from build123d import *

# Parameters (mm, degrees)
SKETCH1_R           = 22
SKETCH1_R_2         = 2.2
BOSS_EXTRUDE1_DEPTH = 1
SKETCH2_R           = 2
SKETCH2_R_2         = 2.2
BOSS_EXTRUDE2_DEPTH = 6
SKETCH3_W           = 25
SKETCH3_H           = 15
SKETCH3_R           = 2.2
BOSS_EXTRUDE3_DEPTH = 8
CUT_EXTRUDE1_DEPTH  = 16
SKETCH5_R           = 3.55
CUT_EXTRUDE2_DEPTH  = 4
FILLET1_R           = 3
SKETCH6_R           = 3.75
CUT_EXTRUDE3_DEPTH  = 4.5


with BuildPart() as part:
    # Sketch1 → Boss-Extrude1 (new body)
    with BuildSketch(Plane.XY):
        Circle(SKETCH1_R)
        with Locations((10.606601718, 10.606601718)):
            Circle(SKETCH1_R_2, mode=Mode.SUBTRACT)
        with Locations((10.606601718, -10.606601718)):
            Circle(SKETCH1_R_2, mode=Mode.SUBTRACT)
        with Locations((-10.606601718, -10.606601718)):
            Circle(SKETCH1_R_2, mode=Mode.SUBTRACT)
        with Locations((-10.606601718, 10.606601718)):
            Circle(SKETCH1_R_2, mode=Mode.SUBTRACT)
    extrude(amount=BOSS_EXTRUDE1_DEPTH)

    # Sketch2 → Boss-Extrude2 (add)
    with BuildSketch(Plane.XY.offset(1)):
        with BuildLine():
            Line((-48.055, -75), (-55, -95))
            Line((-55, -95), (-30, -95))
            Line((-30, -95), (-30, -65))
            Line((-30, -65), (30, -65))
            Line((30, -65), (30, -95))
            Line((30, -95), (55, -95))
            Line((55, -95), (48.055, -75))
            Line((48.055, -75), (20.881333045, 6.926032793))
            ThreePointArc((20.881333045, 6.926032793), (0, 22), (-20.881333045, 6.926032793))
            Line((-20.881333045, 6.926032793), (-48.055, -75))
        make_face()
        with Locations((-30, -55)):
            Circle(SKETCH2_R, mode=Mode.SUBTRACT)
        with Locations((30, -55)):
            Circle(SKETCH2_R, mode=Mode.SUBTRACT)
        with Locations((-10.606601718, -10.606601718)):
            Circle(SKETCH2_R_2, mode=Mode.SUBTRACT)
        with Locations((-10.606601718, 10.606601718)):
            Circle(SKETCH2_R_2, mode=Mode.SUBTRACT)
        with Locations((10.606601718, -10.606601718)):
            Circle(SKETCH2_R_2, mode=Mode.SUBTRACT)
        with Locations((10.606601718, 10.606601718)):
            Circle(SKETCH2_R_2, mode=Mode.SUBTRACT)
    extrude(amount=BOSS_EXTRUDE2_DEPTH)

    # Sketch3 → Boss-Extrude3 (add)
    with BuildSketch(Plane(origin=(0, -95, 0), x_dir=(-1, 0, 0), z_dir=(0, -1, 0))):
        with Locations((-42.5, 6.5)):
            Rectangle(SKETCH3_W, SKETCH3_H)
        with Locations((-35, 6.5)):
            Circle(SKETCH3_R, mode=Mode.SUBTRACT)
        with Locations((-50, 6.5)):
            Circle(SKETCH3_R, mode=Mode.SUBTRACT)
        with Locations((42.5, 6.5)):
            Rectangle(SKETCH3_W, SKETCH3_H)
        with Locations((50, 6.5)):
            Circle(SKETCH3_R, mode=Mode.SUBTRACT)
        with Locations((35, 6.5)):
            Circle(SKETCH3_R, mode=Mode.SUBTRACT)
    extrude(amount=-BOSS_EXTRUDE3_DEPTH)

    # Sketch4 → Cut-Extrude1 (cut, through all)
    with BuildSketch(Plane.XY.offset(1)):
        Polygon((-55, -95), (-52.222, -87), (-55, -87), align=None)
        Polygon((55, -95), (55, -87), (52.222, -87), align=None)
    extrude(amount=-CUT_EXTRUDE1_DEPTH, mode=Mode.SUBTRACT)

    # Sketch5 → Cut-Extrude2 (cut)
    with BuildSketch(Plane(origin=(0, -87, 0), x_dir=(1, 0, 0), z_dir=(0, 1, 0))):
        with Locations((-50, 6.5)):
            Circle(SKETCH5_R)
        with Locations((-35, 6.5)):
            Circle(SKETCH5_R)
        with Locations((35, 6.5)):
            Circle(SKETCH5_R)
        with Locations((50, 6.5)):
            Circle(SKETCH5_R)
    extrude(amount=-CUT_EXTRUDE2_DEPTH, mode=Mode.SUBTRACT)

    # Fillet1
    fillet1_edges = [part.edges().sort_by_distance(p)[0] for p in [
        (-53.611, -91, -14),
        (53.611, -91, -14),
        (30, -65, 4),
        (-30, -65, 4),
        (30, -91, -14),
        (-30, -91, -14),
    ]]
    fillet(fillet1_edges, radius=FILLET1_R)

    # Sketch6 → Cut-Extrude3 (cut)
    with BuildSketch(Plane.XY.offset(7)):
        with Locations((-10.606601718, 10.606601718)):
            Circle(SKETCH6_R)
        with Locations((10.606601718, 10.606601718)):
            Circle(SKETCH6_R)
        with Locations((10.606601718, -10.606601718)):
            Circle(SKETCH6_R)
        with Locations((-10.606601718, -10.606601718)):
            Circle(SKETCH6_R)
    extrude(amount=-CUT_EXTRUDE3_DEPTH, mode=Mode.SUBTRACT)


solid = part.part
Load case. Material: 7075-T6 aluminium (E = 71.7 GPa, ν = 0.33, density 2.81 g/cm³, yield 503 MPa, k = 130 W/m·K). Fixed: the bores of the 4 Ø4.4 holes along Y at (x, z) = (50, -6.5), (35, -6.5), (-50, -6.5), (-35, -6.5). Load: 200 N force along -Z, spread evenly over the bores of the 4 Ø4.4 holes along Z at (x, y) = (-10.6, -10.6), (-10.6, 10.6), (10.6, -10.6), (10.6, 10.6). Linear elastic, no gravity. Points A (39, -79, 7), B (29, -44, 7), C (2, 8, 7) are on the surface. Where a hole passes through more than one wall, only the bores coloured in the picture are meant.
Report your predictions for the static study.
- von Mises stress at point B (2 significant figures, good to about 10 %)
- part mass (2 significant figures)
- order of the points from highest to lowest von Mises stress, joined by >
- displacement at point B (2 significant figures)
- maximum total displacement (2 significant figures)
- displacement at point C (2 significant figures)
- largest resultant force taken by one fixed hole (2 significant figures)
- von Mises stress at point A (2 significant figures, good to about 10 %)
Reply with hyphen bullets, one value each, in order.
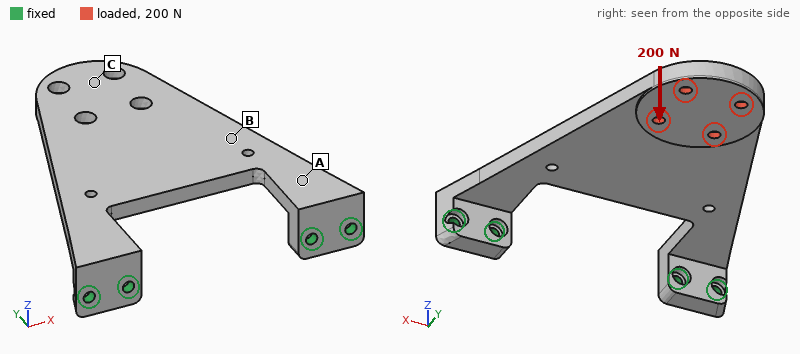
- 26 MPa
- 120 g
- A > B > C
- 0.44 mm
- 1.6 mm
- 1.3 mm
- 110 N
- 66 MPa
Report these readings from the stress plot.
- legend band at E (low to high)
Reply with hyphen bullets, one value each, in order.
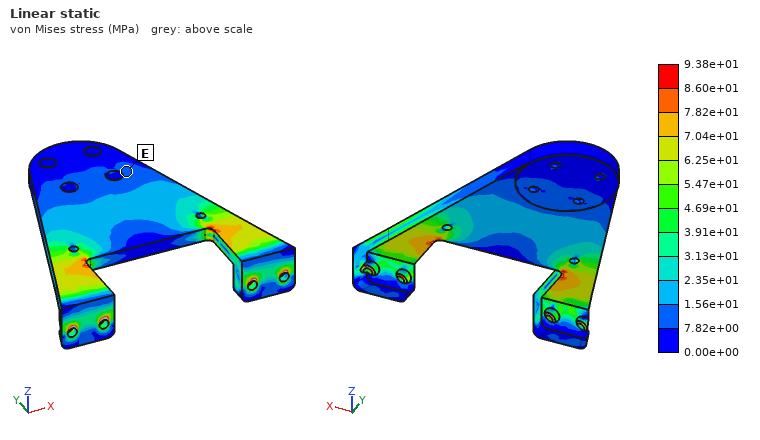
- 7.82e+00 to 1.56e+01 MPa
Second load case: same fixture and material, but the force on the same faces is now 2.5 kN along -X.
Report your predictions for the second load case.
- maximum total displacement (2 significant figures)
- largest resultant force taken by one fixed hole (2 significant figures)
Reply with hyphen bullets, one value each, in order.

- 0.24 mm
- 2.4 kN
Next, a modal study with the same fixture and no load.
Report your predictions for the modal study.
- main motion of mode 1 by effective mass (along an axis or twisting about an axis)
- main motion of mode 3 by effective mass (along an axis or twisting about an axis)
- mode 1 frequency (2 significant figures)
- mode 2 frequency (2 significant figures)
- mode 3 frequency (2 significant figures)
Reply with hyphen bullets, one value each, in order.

- along Z
- along Z
- 320 Hz
- 1800 Hz
- 2000 Hz
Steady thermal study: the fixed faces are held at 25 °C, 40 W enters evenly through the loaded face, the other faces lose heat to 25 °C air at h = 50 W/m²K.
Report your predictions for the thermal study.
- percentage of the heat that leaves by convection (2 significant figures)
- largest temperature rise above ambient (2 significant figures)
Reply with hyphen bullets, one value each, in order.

- 63 %
- 62 K
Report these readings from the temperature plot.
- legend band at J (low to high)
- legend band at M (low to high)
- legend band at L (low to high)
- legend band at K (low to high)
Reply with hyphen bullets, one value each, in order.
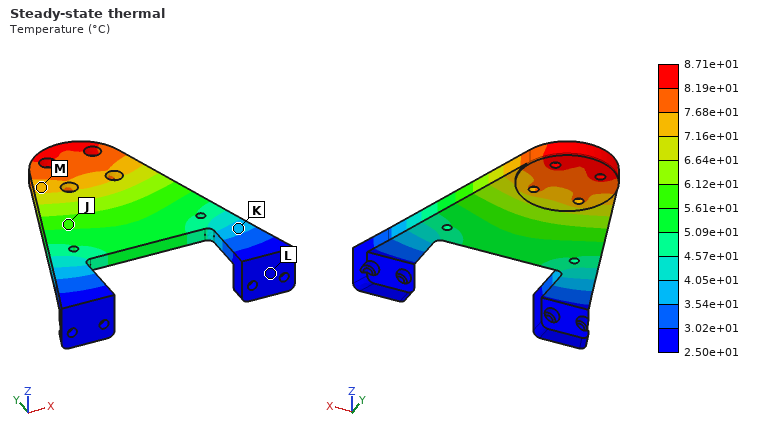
- 5.61e+01 to 6.12e+01 °C
- 7.16e+01 to 7.68e+01 °C
- 2.50e+01 to 3.02e+01 °C
- 3.54e+01 to 4.05e+01 °C
